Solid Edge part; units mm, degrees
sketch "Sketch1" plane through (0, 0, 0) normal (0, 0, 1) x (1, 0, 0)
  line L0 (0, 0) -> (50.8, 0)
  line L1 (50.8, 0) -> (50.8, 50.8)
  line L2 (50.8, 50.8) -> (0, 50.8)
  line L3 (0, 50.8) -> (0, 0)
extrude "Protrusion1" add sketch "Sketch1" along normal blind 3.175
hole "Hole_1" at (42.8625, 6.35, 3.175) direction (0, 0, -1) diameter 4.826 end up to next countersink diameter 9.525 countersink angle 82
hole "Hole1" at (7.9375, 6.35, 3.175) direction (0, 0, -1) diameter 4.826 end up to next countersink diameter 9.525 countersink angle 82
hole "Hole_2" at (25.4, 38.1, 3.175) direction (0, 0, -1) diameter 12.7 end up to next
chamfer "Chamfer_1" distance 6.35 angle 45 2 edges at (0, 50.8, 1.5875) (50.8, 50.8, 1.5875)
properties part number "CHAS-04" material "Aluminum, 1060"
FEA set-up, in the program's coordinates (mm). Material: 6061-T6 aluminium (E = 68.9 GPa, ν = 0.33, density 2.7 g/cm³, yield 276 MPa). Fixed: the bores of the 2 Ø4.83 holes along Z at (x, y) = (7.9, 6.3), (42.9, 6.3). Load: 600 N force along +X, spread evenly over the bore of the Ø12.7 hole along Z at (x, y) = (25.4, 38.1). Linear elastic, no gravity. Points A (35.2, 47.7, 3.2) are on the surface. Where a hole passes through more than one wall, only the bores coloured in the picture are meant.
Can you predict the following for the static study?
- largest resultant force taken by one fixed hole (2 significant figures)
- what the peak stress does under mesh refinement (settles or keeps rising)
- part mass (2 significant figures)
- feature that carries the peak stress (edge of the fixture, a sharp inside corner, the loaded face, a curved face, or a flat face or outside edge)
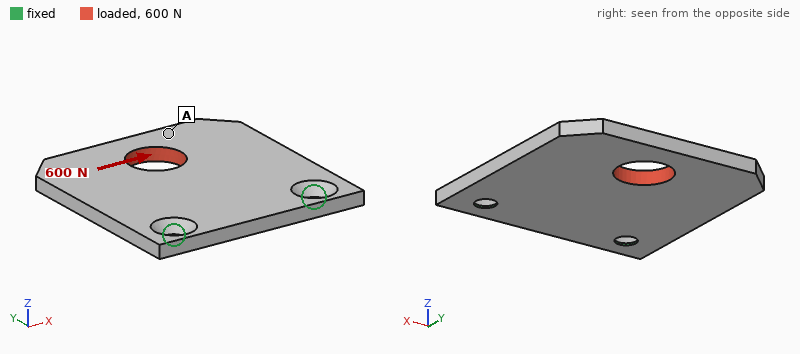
590 N
keeps rising
20 g
edge of the fixture
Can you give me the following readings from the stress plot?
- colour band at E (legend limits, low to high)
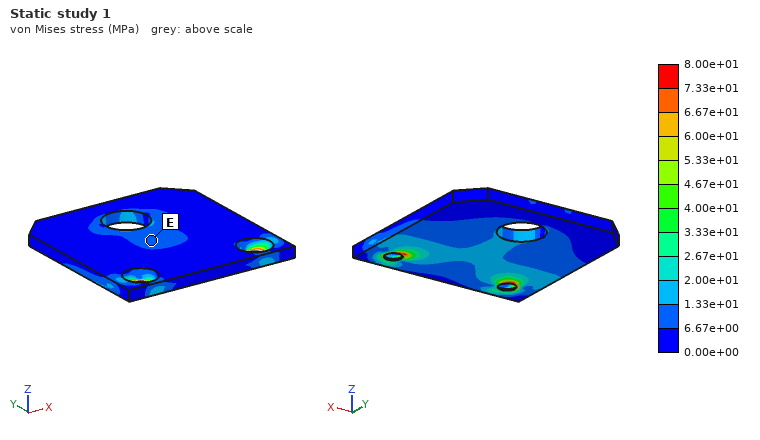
6.67e+00 to 1.33e+01 MPa
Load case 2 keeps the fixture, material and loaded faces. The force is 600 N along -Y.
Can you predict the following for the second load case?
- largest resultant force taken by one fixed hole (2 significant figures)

300 N
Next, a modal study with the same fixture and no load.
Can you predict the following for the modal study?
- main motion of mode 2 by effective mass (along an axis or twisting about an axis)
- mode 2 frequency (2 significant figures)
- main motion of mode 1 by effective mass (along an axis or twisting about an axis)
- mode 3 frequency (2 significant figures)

twisting about Y
2600 Hz
along Z
6200 Hz
